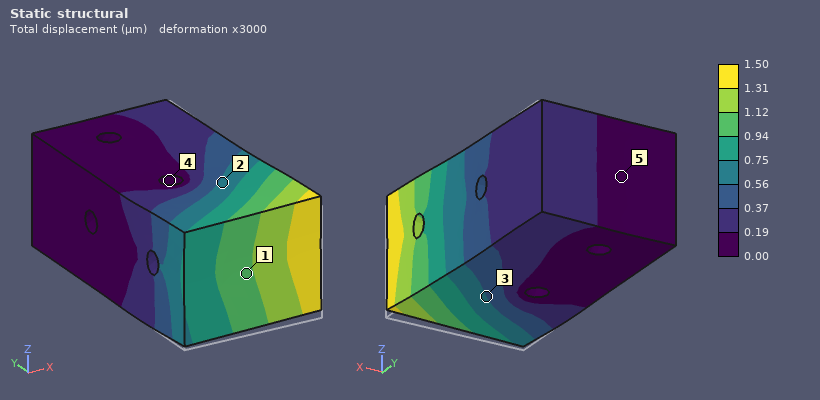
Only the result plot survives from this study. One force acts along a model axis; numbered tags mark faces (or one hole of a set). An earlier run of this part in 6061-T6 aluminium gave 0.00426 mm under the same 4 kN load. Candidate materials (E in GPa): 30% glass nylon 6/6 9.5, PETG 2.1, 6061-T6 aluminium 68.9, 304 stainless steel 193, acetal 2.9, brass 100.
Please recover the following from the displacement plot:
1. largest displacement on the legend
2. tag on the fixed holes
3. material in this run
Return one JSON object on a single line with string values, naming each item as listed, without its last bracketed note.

{"largest displacement on the legend": "1.50 µm", "tag on the fixed holes": "4", "material in this run": "304 stainless steel"}
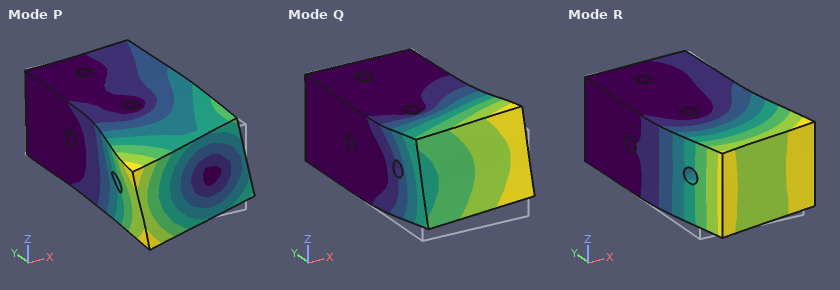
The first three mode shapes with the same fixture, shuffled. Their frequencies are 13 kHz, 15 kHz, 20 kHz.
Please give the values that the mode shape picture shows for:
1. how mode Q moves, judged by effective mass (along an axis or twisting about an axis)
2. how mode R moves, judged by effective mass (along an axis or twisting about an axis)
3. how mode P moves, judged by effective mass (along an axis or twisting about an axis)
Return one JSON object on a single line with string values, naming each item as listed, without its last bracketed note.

{"how mode Q moves, judged by effective mass": "along Z", "how mode R moves, judged by effective mass": "along X", "how mode P moves, judged by effective mass": "twisting about Y"}
